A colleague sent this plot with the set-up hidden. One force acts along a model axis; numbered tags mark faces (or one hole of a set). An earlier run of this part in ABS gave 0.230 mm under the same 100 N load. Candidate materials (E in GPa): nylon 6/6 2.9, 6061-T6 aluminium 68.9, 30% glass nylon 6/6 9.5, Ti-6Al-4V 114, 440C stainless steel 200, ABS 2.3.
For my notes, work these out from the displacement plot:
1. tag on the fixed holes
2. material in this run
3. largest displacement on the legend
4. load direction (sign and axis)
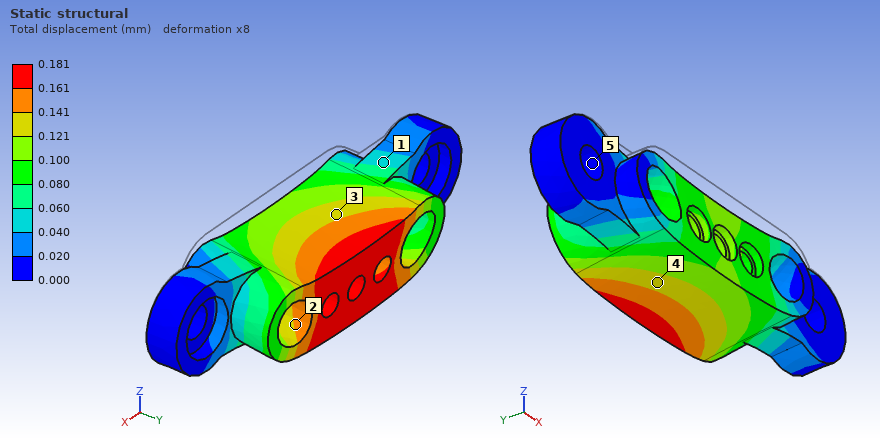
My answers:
5
nylon 6/6
0.181 mm
-Z
